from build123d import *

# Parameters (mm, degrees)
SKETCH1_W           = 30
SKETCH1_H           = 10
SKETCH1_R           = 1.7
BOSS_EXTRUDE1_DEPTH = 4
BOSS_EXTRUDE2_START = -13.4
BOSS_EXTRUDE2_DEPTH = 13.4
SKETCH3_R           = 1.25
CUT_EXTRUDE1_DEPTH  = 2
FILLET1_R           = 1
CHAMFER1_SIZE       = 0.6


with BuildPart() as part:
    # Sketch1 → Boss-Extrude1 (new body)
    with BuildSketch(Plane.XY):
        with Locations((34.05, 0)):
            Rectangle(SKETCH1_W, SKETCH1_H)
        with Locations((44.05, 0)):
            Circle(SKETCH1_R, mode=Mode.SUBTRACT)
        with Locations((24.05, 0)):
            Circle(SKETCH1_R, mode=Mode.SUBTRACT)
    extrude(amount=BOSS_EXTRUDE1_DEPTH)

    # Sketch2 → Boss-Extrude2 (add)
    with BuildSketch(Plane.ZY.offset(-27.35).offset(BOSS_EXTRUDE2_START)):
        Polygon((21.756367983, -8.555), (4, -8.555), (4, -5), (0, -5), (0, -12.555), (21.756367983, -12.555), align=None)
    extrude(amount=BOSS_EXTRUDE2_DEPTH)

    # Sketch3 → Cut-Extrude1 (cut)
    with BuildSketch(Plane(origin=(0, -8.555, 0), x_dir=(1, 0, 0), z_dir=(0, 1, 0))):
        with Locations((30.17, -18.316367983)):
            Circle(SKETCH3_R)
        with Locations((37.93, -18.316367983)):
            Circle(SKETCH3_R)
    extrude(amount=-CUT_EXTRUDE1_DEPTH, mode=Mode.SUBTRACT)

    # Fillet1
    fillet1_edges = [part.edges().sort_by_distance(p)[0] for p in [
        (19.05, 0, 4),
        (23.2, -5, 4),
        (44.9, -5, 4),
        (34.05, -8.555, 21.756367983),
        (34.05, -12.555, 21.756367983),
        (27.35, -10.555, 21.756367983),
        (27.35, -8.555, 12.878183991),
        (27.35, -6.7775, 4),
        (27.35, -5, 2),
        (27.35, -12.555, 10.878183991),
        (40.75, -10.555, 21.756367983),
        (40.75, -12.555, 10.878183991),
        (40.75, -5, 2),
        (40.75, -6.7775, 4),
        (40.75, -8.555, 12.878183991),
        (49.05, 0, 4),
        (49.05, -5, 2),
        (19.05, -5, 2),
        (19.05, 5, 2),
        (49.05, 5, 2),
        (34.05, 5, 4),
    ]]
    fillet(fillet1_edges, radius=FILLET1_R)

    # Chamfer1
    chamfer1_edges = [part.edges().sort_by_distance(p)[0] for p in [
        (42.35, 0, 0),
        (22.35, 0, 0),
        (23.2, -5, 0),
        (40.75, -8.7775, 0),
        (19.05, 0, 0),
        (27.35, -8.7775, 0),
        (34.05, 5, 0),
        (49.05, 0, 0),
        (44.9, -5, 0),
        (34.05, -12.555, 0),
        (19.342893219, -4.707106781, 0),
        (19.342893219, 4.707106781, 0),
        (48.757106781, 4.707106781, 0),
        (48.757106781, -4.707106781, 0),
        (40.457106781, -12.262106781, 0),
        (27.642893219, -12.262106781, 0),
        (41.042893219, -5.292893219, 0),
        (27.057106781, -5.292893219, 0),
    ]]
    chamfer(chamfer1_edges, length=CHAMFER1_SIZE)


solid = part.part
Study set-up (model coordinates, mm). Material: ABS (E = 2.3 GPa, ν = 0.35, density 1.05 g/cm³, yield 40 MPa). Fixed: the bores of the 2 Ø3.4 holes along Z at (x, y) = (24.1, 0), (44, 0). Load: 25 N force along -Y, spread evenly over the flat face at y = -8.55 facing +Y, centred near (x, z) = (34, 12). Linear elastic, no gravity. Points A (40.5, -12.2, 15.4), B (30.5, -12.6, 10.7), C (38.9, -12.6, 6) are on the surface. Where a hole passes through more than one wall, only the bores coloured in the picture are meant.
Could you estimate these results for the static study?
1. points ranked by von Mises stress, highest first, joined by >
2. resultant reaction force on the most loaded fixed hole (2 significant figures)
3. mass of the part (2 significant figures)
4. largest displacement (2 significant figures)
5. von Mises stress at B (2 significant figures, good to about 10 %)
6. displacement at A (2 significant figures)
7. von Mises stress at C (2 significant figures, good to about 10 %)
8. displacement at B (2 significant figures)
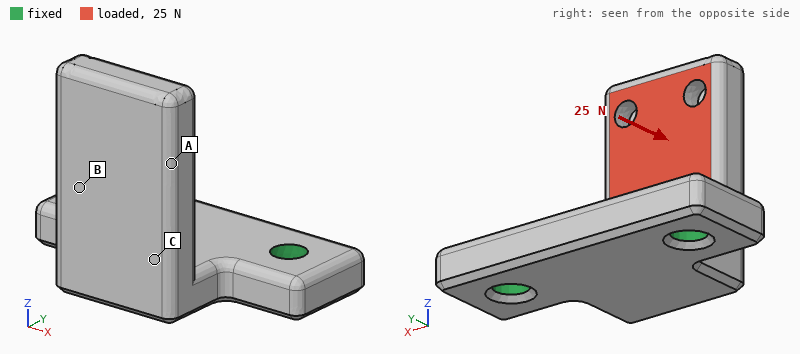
C > B > A
14 N
2.5 g
0.46 mm
2.0 MPa
0.32 mm
4.6 MPa
0.23 mm
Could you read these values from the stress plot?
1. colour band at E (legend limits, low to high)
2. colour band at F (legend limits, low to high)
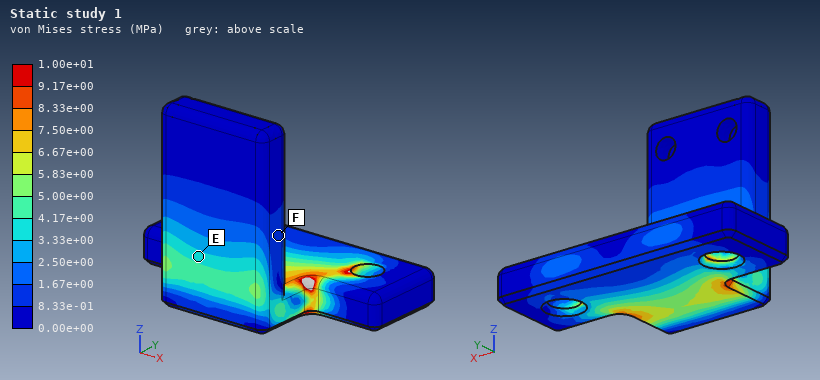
3.33e+00 to 4.17e+00 MPa
8.33e-01 to 1.67e+00 MPa
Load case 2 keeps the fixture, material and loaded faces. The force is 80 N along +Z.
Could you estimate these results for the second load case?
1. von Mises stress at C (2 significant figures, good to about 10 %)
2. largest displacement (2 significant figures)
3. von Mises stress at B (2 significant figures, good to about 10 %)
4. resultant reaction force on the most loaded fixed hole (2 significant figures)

2.6 MPa
0.37 mm
1.8 MPa
40 N
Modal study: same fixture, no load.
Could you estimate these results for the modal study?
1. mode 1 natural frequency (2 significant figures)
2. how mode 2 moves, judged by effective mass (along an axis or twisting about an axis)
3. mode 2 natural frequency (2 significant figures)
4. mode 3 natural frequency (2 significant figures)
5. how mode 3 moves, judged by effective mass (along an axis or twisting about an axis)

1300 Hz
along X
2400 Hz
3800 Hz
along Z
